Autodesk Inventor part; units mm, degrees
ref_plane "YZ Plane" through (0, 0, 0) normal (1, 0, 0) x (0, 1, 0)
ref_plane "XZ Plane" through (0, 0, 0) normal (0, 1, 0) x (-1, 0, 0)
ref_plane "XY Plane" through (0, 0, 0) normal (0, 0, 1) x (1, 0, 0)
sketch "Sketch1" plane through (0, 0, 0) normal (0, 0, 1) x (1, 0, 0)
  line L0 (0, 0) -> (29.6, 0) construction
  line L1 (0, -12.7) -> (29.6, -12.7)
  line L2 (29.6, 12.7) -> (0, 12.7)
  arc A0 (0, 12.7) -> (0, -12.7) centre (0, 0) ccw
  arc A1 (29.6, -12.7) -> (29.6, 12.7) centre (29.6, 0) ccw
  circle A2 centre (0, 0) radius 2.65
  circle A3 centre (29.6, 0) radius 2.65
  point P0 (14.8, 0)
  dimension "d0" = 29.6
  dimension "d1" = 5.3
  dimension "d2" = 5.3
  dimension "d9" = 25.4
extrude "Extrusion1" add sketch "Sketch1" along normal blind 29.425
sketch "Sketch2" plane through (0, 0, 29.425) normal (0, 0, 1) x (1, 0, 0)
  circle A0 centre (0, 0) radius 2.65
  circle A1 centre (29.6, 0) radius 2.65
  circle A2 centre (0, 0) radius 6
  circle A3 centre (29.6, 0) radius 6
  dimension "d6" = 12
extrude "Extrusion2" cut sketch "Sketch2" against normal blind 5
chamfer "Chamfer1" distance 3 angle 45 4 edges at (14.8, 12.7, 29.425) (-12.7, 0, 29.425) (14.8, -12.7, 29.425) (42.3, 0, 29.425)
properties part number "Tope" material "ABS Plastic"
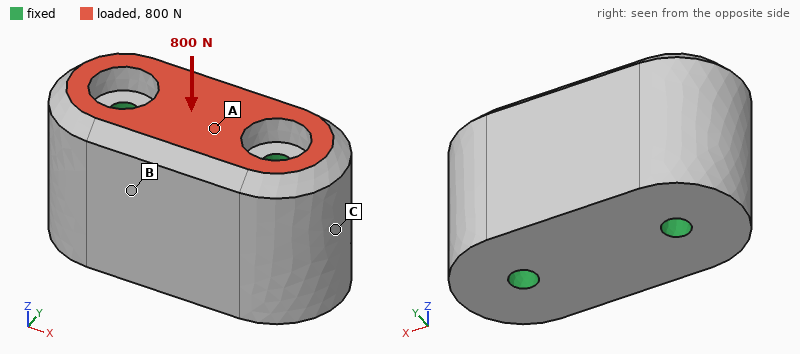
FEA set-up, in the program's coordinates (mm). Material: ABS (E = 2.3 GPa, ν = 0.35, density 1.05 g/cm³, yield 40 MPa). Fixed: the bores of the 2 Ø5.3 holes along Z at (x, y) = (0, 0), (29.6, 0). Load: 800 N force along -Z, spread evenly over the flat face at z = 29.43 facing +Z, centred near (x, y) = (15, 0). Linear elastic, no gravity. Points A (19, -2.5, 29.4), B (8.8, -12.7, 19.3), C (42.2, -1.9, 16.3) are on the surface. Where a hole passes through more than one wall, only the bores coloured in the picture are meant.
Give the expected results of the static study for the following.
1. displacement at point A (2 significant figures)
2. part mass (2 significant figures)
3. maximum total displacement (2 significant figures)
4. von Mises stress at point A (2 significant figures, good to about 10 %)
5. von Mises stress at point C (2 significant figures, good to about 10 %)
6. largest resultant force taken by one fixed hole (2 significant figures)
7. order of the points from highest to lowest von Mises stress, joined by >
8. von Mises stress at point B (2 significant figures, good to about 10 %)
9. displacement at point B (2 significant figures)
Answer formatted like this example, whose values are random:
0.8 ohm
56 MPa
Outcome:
11 µm
36 g
12 µm
0.83 MPa
0.28 MPa
410 N
A > B > C
0.45 MPa
7.5 µm
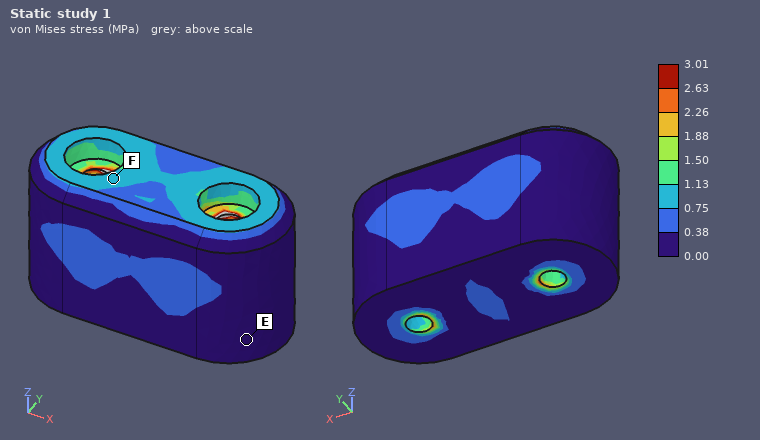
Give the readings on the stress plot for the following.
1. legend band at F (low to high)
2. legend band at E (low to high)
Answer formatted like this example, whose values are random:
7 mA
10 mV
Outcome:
0.75 to 1.13 MPa
0.00 to 0.38 MPa
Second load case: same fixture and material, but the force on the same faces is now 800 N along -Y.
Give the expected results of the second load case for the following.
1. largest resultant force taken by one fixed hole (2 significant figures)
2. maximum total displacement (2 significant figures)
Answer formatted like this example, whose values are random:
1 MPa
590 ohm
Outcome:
400 N
41 µm
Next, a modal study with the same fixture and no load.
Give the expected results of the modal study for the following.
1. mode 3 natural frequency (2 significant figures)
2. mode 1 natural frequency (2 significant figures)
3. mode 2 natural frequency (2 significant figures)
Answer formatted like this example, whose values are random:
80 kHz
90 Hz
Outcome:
11 kHz
9400 Hz
11 kHz
